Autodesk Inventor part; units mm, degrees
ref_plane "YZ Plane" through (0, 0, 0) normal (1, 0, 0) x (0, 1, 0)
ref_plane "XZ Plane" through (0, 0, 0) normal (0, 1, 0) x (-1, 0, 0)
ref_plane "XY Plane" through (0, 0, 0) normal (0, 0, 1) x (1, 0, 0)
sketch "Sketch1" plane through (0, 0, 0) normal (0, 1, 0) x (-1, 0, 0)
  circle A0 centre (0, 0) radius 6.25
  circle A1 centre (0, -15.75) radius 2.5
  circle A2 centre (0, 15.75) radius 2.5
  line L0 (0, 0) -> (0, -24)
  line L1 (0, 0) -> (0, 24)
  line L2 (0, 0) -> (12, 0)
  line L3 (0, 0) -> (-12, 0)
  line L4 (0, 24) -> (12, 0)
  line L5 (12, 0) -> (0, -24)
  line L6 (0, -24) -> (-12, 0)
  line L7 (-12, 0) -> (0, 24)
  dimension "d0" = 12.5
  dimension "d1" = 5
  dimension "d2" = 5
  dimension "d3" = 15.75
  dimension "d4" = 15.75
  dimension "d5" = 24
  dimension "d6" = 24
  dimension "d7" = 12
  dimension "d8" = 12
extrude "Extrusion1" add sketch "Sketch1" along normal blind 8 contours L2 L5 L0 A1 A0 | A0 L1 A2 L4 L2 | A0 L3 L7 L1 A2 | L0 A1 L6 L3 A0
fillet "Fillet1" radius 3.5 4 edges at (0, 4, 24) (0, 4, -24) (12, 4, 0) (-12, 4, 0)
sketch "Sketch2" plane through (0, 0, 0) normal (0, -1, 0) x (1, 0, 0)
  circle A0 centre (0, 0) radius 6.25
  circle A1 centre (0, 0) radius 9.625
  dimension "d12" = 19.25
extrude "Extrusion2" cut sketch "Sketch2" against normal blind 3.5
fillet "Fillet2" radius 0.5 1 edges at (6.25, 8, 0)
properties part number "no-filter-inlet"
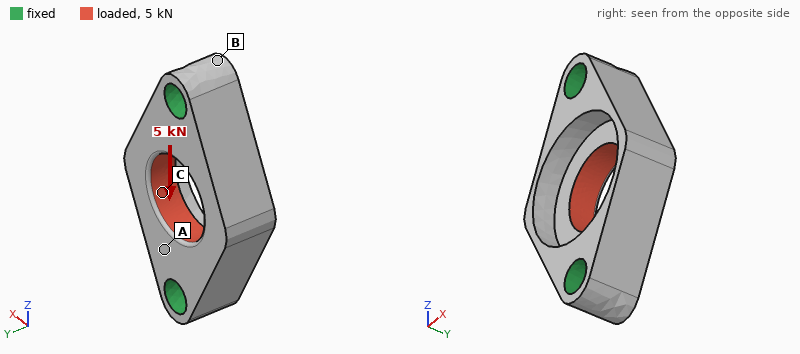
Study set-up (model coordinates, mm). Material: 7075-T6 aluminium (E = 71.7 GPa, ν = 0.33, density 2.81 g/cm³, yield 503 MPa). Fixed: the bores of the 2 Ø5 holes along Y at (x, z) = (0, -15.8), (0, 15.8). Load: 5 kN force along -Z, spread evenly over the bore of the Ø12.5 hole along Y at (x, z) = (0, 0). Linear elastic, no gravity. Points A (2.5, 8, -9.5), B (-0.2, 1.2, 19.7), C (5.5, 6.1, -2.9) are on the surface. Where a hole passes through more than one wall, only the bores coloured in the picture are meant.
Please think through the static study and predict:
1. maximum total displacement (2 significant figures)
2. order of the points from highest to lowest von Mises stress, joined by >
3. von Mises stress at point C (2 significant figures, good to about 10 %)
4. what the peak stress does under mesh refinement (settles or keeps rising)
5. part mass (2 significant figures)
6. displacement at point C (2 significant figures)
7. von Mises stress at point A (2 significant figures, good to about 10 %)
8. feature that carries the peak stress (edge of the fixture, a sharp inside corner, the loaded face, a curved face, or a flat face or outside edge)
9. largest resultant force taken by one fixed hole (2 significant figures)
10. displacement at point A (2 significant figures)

10 µm
C > A > B
74 MPa
keeps rising
7.1 g
9.0 µm
42 MPa
edge of the fixture
2.5 kN
3.4 µm
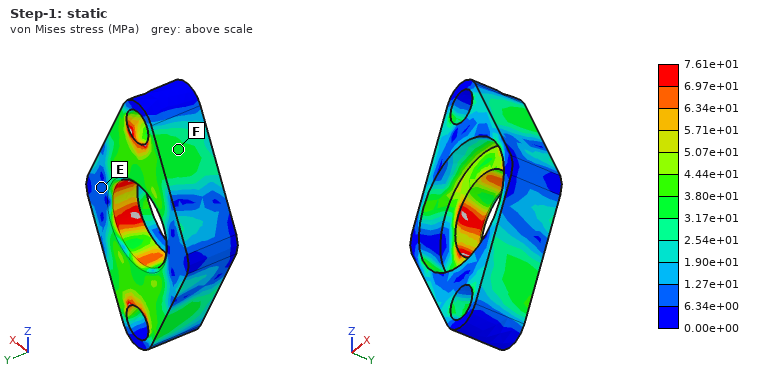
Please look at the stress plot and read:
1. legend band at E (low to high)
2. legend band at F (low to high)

6.34e+00 to 1.27e+01 MPa
3.17e+01 to 3.80e+01 MPa
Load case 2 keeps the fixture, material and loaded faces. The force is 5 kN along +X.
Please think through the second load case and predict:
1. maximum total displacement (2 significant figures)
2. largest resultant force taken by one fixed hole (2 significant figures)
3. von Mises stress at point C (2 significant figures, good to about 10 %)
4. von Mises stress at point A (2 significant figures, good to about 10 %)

24 µm
2.5 kN
50 MPa
71 MPa
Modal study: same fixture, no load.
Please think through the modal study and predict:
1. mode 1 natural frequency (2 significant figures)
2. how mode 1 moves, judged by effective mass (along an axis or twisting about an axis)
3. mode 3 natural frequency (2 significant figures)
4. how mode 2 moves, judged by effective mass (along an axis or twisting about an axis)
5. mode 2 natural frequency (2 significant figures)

28 kHz
twisting about Z
47 kHz
along Y
29 kHz
